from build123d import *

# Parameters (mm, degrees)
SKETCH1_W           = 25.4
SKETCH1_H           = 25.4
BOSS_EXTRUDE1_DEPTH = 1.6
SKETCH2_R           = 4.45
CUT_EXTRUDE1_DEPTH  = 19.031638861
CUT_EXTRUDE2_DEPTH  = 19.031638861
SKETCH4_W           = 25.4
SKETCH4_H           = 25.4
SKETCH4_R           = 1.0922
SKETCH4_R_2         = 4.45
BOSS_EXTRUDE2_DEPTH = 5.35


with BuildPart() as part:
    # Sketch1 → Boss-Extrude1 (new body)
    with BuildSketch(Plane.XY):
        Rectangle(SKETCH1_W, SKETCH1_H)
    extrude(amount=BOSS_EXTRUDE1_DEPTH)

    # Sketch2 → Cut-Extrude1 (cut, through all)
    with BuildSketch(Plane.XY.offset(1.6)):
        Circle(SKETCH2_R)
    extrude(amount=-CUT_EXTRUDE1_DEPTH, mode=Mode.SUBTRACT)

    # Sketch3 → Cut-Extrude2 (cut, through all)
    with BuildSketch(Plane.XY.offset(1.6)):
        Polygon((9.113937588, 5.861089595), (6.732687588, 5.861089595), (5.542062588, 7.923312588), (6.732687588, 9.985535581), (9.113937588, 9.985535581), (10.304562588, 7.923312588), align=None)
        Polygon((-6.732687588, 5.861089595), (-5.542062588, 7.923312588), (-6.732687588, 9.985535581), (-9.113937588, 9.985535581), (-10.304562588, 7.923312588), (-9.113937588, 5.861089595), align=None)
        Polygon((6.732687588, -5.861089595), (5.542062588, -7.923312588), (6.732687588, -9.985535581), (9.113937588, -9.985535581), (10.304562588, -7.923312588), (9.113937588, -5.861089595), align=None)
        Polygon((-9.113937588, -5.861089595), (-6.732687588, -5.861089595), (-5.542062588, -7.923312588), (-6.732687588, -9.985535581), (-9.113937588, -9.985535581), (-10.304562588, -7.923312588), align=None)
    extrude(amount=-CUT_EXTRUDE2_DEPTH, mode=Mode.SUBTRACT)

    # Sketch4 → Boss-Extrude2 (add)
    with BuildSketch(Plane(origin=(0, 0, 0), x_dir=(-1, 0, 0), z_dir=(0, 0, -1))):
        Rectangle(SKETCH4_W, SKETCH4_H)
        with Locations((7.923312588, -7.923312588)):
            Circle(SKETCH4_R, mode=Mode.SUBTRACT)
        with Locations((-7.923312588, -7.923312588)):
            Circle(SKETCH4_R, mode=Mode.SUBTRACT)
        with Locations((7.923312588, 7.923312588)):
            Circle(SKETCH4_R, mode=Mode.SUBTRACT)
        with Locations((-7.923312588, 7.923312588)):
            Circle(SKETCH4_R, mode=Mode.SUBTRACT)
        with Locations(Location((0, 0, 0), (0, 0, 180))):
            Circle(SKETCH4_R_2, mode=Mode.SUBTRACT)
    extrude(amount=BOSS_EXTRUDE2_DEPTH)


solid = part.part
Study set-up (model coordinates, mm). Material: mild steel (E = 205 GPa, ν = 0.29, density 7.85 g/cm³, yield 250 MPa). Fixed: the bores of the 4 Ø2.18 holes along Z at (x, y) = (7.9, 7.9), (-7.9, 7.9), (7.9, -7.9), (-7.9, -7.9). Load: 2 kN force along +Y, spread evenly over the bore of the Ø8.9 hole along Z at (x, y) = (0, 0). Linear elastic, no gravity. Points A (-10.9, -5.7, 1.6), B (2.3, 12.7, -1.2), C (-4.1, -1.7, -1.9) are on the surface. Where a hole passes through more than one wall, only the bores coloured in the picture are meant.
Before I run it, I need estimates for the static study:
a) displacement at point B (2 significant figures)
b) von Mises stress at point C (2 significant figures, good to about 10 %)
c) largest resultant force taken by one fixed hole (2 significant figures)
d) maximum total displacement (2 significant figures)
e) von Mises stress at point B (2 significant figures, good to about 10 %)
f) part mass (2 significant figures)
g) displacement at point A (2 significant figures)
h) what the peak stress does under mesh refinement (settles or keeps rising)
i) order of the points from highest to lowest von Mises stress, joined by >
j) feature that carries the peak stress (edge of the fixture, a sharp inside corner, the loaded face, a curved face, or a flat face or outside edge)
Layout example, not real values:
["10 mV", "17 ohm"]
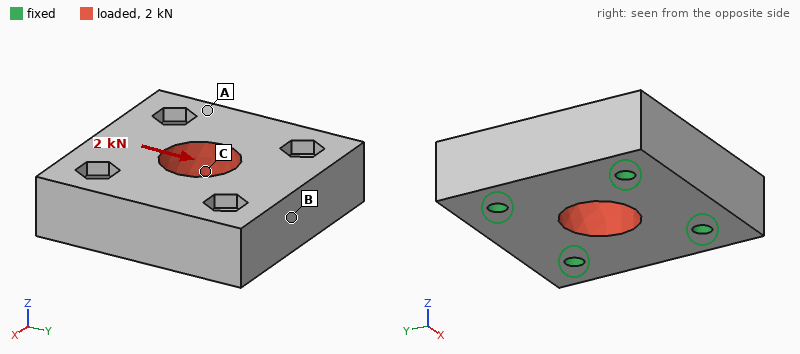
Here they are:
["0.46 µm", "19 MPa", "520 N", "0.75 µm", "8.3 MPa", "30 g", "0.12 µm", "keeps rising", "C > B > A", "edge of the fixture"]
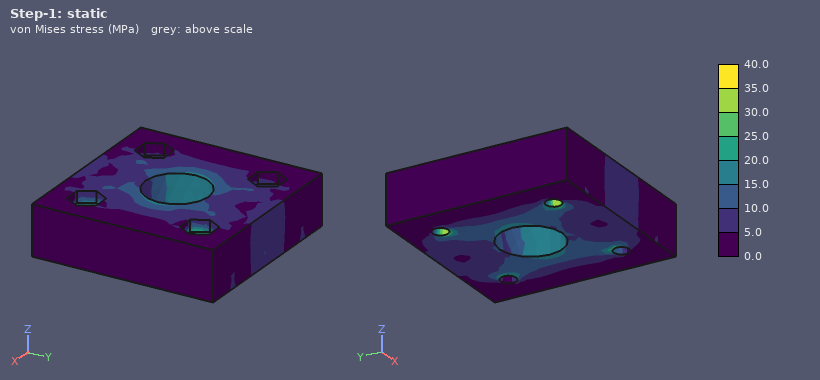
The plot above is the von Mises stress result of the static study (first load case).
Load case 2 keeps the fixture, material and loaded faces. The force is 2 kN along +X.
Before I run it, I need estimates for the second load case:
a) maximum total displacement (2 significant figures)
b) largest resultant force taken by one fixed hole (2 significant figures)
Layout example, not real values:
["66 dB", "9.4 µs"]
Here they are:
["0.75 µm", "520 N"]
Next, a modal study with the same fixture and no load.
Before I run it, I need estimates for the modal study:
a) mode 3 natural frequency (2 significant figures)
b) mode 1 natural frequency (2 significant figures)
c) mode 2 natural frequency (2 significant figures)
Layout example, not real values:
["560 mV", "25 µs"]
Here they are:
["67 kHz", "61 kHz", "62 kHz"]
